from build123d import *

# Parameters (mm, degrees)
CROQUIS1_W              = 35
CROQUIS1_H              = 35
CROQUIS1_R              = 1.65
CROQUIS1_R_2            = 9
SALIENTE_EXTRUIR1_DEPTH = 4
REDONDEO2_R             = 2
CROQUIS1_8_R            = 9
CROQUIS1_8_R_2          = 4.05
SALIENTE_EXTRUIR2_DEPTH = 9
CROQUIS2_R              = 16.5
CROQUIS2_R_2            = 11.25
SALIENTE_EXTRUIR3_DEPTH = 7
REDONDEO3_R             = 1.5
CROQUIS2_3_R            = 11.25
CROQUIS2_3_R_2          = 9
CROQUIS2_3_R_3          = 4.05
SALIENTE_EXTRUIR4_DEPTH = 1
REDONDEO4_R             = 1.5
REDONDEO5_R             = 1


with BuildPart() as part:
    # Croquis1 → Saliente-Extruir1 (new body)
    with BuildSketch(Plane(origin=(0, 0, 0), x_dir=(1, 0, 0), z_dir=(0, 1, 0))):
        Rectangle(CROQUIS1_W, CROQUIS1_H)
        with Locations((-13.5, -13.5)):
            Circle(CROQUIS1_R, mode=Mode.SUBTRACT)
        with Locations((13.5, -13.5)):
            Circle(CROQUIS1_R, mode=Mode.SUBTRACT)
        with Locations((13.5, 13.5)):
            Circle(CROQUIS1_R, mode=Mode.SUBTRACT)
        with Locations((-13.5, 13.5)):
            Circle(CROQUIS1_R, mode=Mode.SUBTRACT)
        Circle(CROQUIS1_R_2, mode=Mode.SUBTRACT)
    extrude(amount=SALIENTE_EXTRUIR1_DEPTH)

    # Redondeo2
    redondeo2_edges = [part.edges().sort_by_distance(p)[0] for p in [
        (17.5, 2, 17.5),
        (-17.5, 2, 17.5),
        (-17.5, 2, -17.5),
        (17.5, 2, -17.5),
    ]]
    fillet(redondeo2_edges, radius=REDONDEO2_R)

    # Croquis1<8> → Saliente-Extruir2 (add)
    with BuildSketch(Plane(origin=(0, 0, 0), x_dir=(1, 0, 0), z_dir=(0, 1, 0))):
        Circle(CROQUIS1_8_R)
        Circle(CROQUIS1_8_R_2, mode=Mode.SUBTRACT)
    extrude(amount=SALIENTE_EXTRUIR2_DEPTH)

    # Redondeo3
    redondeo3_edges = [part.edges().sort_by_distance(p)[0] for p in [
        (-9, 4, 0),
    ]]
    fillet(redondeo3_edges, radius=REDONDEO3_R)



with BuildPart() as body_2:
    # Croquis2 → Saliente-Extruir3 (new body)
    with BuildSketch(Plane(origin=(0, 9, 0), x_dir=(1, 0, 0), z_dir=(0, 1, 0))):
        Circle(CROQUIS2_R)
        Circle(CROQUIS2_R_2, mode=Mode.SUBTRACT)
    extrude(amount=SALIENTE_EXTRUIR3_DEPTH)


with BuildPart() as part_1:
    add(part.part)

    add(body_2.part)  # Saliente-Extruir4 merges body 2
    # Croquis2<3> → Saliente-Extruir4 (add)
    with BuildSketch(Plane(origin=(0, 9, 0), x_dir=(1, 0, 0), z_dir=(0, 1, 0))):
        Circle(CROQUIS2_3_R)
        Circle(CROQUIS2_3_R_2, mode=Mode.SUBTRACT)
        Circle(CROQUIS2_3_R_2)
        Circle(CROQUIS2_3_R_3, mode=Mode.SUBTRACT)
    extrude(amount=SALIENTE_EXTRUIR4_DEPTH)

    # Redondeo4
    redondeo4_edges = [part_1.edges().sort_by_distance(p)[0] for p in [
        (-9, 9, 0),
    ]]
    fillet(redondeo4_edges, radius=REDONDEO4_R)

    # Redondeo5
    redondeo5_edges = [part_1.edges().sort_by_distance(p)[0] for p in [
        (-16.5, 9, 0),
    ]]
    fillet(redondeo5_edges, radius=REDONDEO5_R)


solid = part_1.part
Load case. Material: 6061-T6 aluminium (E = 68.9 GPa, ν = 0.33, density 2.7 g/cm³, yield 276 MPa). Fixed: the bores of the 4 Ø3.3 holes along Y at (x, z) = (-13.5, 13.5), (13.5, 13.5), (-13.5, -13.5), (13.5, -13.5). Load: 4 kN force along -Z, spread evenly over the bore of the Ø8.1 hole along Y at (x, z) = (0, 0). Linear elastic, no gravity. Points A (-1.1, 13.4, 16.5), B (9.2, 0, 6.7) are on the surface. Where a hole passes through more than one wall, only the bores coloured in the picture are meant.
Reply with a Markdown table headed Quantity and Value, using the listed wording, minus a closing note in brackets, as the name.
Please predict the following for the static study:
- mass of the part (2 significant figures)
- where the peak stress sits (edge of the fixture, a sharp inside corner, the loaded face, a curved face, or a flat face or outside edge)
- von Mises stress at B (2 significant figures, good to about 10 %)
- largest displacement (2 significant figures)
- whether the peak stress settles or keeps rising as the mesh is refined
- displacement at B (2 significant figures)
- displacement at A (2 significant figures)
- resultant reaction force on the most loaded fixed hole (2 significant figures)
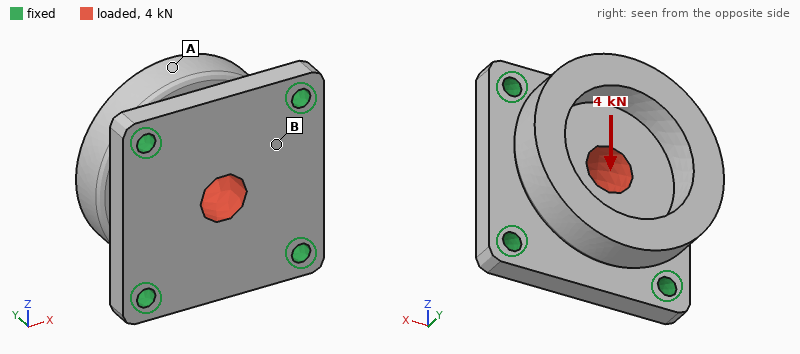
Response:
| Quantity | Value |
|---|---|
| mass of the part | 25 g |
| where the peak stress sits | edge of the fixture |
| von Mises stress at B | 17 MPa |
| largest displacement | 20 µm |
| whether the peak stress settles or keeps rising as the mesh is refined | keeps rising |
| displacement at B | 4.6 µm |
| displacement at A | 19 µm |
| resultant reaction force on the most loaded fixed hole | 1.1 kN |
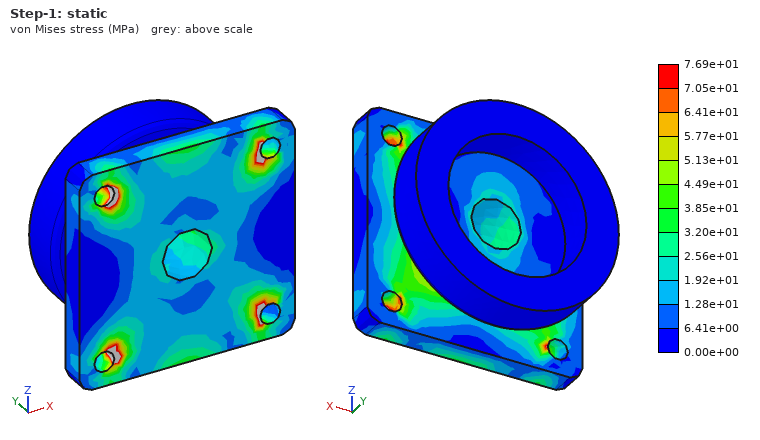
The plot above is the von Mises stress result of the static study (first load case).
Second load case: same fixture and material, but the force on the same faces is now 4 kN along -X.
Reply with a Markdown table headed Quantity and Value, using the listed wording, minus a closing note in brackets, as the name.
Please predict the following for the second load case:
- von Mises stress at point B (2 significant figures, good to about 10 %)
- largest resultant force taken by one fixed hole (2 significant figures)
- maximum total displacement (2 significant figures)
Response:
| Quantity | Value |
|---|---|
| von Mises stress at point B | 17 MPa |
| largest resultant force taken by one fixed hole | 1.1 kN |
| maximum total displacement | 20 µm |
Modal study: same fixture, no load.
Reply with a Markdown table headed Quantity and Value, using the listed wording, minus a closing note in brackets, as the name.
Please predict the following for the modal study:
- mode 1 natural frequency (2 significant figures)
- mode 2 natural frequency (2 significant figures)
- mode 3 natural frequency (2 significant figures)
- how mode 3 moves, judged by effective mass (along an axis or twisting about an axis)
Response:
| Quantity | Value |
|---|---|
| mode 1 natural frequency | 9000 Hz |
| mode 2 natural frequency | 9000 Hz |
| mode 3 natural frequency | 12 kHz |
| how mode 3 moves, judged by effective mass | along Y |
